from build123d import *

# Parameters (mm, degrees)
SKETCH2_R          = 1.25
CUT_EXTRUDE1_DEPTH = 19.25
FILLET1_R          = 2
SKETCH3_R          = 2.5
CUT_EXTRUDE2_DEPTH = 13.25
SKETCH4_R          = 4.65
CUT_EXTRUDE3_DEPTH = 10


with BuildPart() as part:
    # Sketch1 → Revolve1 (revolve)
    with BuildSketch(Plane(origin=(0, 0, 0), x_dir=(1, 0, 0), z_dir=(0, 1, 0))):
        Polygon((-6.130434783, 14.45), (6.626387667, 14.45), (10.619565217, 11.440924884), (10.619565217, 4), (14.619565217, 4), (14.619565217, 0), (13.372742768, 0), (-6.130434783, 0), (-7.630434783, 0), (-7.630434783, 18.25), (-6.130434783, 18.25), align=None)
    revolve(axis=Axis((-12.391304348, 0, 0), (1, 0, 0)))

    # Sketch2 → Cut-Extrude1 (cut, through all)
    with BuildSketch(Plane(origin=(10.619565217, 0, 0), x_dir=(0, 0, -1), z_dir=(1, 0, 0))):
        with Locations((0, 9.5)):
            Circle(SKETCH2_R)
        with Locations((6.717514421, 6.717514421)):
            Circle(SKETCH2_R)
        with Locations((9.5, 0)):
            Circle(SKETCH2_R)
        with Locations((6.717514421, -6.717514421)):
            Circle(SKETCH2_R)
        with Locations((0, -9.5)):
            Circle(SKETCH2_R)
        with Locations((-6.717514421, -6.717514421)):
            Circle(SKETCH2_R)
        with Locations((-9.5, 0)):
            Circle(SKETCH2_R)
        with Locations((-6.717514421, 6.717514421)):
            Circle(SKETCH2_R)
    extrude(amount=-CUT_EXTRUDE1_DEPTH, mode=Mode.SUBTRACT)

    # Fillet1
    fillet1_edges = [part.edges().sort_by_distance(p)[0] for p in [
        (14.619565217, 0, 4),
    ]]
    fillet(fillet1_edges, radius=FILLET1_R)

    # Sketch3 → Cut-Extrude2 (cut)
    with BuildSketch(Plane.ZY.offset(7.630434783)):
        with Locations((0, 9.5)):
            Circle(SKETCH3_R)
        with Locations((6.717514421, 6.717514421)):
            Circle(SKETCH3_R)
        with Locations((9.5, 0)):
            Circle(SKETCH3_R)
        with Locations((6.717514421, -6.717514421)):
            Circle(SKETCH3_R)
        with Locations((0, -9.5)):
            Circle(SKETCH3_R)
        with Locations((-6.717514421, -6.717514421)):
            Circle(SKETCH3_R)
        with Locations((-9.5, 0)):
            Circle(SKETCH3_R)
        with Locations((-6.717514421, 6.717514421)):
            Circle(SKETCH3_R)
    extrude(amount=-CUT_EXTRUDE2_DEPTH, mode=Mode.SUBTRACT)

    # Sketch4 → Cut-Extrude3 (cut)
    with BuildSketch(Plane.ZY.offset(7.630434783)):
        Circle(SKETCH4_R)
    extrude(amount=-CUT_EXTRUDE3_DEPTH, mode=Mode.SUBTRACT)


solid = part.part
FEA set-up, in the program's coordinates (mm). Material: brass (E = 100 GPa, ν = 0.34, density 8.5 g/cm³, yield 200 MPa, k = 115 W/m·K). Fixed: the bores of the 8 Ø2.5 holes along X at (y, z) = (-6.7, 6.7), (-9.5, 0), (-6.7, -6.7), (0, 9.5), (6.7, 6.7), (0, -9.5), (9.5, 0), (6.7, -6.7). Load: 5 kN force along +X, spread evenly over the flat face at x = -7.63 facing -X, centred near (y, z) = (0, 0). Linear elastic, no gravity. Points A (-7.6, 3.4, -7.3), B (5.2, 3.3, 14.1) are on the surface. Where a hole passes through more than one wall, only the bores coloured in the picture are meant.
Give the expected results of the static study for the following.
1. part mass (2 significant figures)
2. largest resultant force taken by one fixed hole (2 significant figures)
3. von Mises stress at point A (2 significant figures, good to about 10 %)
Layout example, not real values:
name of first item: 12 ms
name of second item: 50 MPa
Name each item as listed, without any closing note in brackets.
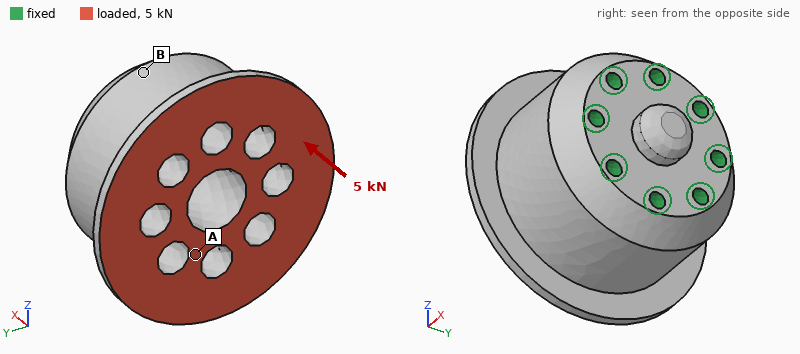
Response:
part mass: 79 g
largest resultant force taken by one fixed hole: 630 N
von Mises stress at point A: 19 MPa
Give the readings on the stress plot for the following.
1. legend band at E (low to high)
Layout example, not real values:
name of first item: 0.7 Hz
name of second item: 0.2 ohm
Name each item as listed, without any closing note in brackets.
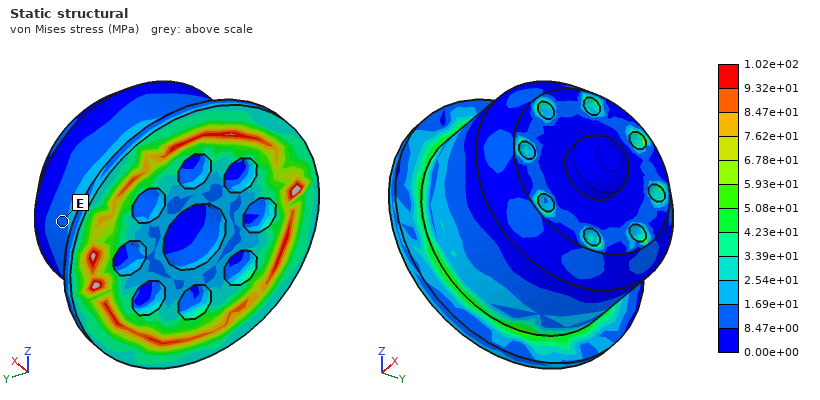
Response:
legend band at E: 8.47e+00 to 1.69e+01 MPa
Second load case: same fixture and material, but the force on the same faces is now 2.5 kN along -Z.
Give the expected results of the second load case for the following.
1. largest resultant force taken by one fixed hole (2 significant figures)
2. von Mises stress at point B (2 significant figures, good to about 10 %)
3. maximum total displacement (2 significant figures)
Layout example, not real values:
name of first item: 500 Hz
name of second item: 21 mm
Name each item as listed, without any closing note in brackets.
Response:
largest resultant force taken by one fixed hole: 880 N
von Mises stress at point B: 8.7 MPa
maximum total displacement: 13 µm
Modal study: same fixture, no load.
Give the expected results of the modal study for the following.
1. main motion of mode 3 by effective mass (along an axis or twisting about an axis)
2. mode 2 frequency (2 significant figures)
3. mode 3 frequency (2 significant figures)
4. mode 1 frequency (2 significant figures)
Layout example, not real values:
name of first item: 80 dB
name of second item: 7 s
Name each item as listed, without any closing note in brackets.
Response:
main motion of mode 3 by effective mass: twisting about X
mode 2 frequency: 18 kHz
mode 3 frequency: 25 kHz
mode 1 frequency: 18 kHz
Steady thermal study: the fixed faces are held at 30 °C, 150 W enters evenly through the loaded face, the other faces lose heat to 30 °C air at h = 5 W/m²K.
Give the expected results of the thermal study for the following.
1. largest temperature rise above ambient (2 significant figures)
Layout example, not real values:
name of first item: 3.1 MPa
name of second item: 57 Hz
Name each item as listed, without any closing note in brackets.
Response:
largest temperature rise above ambient: 62 K
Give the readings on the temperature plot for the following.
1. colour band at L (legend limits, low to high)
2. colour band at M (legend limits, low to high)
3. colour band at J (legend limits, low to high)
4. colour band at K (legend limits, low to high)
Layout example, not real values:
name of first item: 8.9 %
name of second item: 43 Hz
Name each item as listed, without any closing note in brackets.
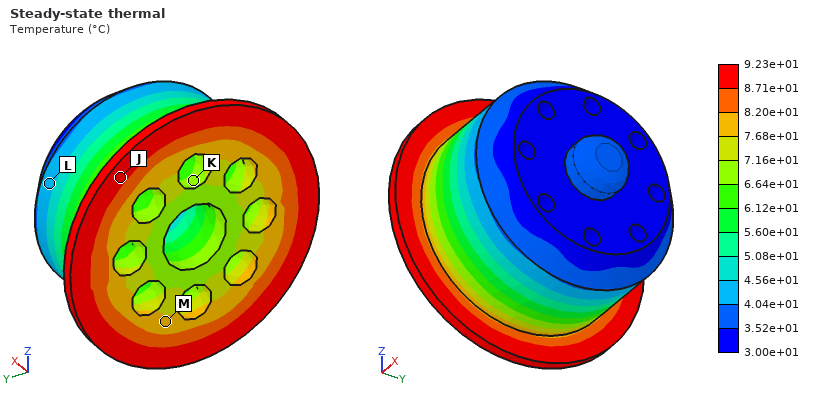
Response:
colour band at L: 4.04e+01 to 4.56e+01 °C
colour band at M: 7.68e+01 to 8.20e+01 °C
colour band at J: 8.71e+01 to 9.23e+01 °C
colour band at K: 6.64e+01 to 7.16e+01 °C
